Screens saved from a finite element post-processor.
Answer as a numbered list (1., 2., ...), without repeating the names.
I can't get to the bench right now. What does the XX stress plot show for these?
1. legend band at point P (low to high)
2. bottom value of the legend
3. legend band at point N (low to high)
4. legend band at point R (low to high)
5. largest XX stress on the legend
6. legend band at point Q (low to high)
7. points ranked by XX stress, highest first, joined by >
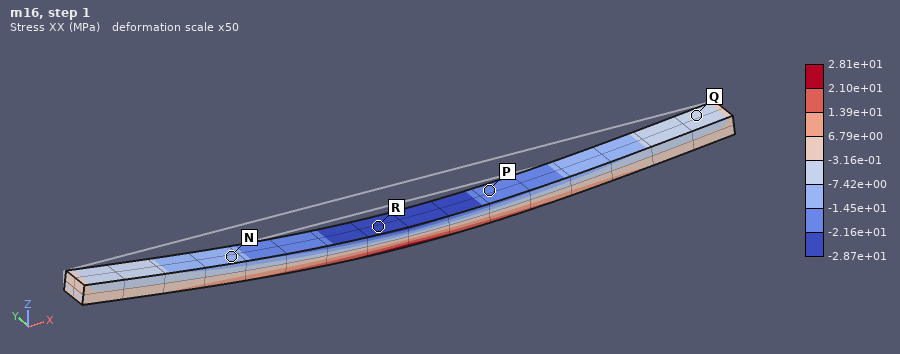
1. -2.16e+01 to -1.45e+01 MPa
2. -2.87e+01 MPa
3. -1.45e+01 to -7.42e+00 MPa
4. -2.87e+01 to -2.16e+01 MPa
5. 2.81e+01 MPa
6. -7.42e+00 to -3.16e-01 MPa
7. Q > N > P > R
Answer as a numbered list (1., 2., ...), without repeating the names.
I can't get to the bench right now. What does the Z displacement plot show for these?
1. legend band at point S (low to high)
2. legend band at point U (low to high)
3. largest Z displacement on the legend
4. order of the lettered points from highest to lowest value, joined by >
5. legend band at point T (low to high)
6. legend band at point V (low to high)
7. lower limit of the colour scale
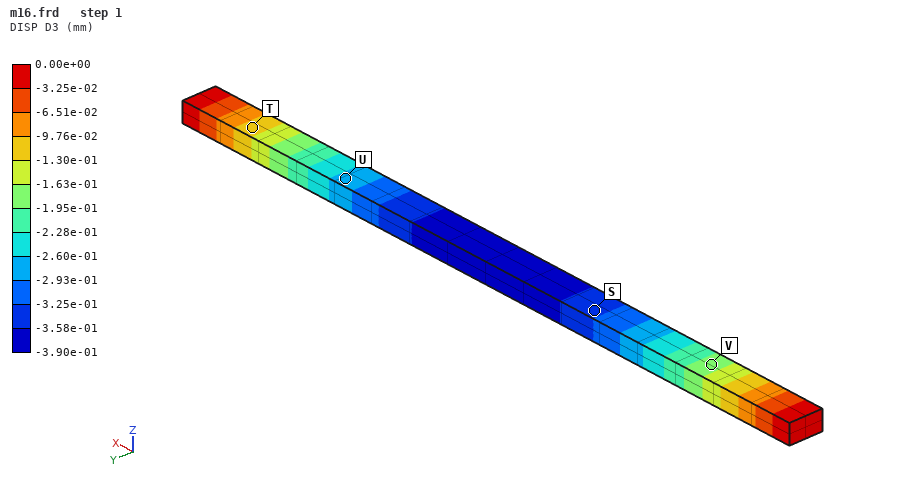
1. -3.58e-01 to -3.25e-01 mm
2. -2.93e-01 to -2.60e-01 mm
3. 0.00e+00 mm
4. T > V > U > S
5. -1.30e-01 to -9.76e-02 mm
6. -1.95e-01 to -1.63e-01 mm
7. -3.90e-01 mm
